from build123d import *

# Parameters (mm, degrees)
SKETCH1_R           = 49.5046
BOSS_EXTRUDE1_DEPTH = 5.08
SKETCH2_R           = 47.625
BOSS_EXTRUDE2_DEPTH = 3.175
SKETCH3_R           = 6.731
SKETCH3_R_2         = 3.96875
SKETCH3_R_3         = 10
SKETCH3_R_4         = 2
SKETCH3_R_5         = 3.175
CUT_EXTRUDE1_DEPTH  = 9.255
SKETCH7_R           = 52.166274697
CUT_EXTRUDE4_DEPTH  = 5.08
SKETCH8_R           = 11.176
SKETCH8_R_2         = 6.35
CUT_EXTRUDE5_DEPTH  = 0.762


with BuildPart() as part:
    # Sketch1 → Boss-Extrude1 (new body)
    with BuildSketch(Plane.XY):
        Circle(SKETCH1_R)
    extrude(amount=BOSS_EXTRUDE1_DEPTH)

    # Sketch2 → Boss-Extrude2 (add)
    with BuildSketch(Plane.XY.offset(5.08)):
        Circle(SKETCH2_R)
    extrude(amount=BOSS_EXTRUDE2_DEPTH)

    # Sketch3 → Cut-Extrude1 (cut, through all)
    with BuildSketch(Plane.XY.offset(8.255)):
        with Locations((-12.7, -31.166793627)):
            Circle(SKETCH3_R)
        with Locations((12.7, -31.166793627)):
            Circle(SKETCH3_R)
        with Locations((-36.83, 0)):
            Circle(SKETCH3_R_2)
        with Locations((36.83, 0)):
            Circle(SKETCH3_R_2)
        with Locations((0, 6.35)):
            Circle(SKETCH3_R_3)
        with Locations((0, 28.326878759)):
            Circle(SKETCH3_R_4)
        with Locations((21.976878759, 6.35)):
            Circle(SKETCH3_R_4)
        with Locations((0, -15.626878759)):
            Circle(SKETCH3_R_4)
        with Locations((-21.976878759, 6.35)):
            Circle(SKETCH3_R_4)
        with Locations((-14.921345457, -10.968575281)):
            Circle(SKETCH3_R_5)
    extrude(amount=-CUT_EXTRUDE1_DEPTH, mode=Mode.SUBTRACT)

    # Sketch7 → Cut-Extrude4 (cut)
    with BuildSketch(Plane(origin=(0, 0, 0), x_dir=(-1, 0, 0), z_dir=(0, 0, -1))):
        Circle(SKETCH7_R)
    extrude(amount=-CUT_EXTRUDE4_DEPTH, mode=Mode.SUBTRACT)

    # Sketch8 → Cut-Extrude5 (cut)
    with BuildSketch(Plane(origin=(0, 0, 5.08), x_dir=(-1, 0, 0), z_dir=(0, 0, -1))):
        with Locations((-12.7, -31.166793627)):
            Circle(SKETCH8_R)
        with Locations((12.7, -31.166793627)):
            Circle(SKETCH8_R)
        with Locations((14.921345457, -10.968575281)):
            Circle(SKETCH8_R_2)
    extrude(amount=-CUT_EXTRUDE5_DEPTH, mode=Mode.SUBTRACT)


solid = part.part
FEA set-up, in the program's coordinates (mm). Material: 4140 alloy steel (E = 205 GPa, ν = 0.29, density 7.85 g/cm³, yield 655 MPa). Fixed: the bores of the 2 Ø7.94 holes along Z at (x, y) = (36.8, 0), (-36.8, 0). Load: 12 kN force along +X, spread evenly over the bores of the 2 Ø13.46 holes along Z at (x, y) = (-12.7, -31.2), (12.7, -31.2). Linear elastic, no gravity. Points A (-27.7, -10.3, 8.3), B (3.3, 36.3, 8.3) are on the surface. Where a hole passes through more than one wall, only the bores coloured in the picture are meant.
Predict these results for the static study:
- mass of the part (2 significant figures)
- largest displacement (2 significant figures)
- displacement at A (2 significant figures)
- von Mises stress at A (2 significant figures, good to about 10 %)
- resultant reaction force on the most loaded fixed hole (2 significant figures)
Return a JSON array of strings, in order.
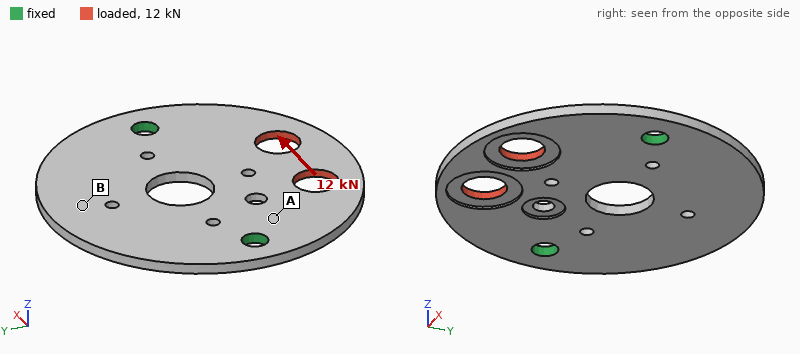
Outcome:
["150 g", "42 µm", "8.4 µm", "110 MPa", "7.8 kN"]
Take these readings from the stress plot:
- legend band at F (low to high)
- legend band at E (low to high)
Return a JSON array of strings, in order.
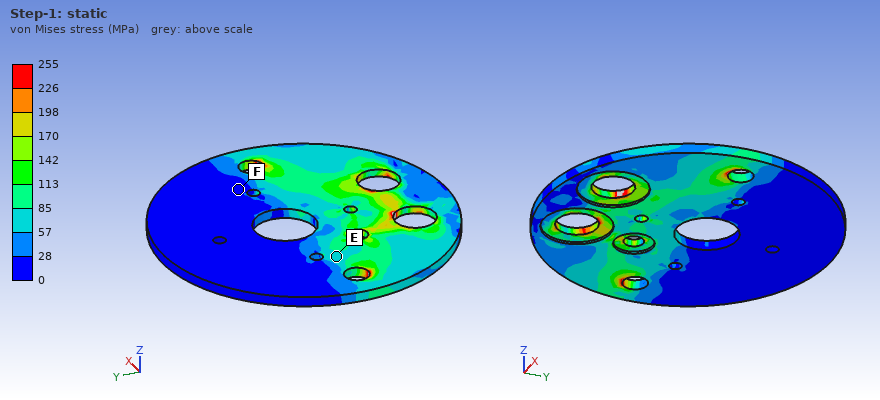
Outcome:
["0 to 28 MPa", "57 to 85 MPa"]
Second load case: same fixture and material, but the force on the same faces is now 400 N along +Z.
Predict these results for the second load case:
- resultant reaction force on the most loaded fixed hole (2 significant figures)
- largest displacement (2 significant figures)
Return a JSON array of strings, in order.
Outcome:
["210 N", "0.26 mm"]
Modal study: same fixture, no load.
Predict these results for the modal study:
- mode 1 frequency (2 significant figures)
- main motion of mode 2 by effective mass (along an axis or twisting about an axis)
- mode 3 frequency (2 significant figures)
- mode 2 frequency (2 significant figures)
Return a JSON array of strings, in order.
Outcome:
["1200 Hz", "along Z", "3100 Hz", "1400 Hz"]
